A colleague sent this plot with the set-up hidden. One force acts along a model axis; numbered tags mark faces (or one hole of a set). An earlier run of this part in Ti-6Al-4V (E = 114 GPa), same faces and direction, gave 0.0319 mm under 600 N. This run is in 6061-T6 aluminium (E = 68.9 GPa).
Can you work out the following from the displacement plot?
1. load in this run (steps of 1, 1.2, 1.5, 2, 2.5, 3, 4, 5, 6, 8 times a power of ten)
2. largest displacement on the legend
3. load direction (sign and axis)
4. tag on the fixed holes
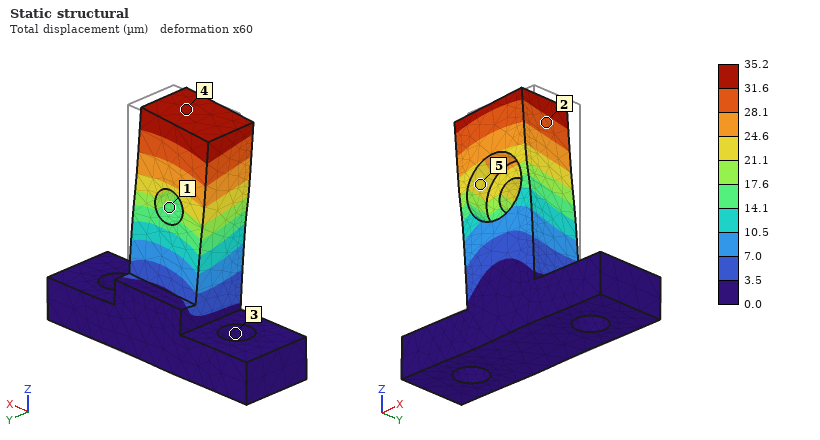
400 N
35.2 µm
-X
3
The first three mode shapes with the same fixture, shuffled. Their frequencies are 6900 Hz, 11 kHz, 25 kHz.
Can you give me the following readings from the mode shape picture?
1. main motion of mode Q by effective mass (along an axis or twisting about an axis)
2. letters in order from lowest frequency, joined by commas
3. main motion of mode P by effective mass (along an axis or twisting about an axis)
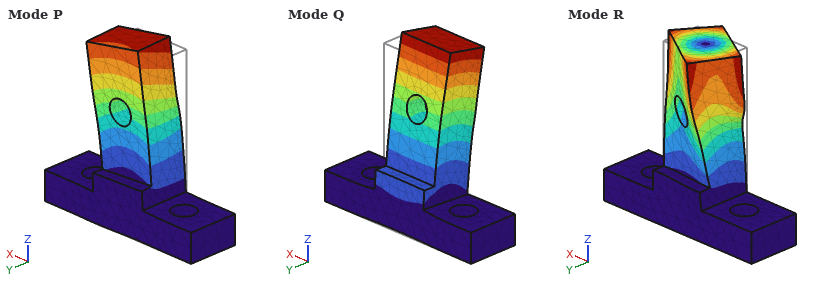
along Y
Q, P, R
along X
